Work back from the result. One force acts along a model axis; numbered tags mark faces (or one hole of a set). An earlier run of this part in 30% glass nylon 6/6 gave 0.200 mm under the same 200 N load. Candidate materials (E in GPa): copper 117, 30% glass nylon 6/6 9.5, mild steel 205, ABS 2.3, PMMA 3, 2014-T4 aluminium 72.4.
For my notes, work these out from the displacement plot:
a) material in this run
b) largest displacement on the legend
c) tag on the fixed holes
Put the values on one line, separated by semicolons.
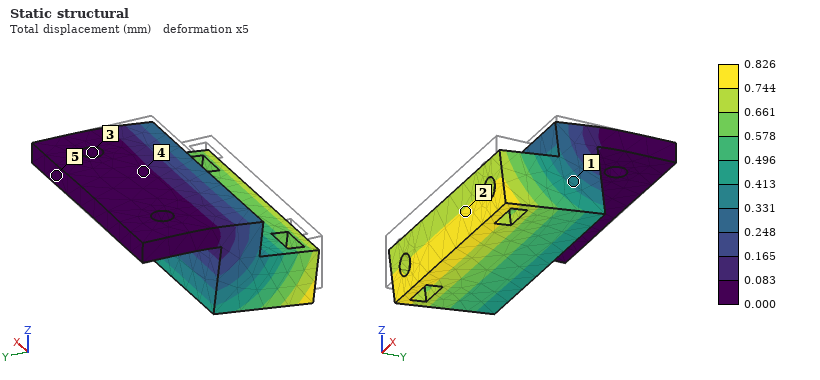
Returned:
ABS; 0.826 mm; 3
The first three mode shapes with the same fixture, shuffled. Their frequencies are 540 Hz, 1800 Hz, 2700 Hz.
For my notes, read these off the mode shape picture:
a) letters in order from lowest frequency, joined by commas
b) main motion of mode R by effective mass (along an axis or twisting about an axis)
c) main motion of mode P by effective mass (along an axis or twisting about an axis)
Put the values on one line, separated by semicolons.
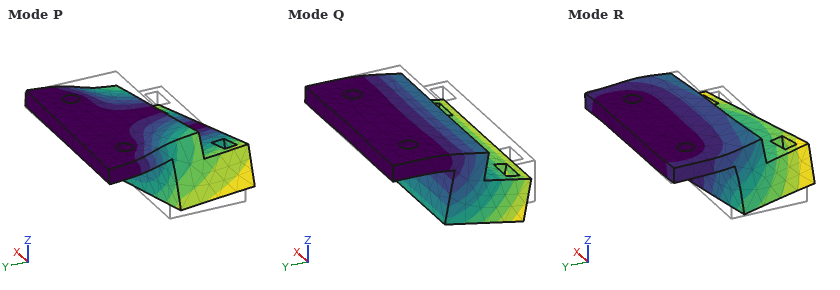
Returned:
Q, P, R; along X; along X
